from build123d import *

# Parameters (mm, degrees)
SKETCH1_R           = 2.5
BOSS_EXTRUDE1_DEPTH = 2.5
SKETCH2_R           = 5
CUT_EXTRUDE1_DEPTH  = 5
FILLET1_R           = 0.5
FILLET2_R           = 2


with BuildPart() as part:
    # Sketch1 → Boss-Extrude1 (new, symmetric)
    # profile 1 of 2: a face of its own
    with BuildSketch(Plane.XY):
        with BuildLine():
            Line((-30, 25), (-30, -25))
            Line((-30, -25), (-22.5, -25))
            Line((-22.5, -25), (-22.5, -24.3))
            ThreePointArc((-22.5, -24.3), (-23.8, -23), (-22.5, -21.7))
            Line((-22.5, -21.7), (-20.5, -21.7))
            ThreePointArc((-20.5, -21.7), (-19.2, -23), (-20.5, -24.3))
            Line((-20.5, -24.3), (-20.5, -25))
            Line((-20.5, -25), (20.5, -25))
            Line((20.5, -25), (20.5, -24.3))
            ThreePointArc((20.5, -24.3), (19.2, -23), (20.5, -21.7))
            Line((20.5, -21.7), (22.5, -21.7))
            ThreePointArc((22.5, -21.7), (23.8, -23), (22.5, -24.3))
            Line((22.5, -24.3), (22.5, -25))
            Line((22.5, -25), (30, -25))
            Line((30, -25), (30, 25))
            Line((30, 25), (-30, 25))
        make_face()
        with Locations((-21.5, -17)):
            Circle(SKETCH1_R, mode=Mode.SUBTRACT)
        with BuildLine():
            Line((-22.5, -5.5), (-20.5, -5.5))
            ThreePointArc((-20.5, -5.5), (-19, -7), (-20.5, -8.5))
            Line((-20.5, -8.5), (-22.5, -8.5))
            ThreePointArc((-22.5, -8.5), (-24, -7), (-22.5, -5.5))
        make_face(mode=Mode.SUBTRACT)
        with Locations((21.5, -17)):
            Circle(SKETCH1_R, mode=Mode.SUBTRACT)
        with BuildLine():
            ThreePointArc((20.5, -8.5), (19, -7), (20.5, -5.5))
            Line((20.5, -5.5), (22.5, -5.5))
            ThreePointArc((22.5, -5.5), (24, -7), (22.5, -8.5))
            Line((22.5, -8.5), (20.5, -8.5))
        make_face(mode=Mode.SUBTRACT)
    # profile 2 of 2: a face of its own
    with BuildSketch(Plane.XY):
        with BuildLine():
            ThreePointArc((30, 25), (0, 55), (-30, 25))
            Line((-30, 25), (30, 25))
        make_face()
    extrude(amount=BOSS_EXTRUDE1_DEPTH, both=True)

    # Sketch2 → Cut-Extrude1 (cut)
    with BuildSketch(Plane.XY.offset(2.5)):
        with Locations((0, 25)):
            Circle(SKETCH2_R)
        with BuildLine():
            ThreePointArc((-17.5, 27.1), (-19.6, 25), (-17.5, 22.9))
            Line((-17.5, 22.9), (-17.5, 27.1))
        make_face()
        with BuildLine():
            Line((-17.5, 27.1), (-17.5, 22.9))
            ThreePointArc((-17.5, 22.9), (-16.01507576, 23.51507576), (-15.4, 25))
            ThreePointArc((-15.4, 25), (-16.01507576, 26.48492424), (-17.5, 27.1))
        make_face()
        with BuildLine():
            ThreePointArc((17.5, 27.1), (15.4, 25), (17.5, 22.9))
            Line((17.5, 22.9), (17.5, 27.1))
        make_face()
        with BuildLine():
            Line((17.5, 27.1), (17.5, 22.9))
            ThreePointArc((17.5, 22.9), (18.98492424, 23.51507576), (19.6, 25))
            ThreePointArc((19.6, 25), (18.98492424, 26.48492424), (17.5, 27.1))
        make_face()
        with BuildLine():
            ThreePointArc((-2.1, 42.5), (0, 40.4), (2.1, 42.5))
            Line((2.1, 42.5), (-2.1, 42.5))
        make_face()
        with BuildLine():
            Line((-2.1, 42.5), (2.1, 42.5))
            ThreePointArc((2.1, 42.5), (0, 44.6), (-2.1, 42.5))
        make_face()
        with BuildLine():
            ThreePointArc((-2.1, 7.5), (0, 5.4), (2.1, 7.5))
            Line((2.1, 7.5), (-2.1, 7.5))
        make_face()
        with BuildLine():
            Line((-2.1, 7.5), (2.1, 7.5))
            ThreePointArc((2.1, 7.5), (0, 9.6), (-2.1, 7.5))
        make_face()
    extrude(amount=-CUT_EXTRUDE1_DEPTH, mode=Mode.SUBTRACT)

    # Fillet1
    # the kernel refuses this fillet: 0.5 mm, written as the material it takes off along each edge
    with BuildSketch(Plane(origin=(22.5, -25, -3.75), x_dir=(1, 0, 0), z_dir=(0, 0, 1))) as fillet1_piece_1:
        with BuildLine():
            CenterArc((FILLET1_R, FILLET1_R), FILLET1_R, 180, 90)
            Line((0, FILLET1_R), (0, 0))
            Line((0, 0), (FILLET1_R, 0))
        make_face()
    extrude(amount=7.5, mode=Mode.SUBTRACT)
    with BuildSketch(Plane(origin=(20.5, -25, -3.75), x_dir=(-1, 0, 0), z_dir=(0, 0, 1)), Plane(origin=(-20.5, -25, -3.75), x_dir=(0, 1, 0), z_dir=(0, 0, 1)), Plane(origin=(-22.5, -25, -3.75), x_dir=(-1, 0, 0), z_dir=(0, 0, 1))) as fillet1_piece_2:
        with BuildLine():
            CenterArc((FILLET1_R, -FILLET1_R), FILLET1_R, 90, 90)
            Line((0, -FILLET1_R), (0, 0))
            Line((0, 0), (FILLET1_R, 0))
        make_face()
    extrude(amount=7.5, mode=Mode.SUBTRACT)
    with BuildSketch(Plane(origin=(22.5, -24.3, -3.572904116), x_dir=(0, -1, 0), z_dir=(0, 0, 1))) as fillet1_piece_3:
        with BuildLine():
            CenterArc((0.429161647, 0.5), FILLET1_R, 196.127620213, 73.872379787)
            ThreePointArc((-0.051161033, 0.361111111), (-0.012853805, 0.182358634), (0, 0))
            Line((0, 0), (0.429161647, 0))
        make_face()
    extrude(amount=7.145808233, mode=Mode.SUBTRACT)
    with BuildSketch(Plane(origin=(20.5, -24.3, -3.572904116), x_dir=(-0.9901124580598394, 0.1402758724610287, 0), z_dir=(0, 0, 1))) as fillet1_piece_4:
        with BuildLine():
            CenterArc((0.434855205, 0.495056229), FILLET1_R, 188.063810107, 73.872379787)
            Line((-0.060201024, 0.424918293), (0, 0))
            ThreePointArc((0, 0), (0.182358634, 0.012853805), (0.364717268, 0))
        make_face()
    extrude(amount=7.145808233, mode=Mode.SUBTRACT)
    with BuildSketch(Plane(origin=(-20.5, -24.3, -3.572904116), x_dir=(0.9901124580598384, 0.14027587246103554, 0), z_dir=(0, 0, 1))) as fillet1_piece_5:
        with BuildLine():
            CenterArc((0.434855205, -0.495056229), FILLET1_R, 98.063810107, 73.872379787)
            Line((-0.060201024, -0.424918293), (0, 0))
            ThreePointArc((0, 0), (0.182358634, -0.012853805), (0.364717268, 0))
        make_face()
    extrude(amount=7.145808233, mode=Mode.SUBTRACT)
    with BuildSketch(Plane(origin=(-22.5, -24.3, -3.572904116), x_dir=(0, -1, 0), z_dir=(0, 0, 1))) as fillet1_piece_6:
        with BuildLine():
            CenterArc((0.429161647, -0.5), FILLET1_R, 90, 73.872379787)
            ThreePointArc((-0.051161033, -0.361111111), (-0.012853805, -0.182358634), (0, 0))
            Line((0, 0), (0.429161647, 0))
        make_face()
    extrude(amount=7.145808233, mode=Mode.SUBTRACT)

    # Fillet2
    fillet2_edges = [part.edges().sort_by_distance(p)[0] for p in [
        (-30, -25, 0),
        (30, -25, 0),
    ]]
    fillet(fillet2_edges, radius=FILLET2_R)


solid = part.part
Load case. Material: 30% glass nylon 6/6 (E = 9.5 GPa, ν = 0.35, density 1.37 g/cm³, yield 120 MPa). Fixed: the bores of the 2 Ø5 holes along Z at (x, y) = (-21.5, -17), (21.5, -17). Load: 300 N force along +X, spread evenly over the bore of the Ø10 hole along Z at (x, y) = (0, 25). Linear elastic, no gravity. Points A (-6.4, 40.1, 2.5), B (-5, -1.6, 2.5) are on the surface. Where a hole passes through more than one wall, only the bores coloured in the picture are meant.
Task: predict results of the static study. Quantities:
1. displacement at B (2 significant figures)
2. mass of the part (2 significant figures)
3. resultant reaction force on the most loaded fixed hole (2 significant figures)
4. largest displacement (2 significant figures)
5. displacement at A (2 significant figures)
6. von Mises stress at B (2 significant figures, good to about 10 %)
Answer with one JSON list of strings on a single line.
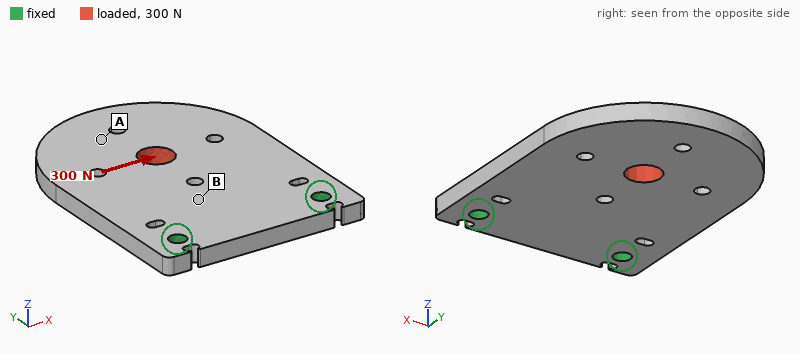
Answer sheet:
["8.6 µm", "29 g", "310 N", "41 µm", "36 µm", "2.5 MPa"]
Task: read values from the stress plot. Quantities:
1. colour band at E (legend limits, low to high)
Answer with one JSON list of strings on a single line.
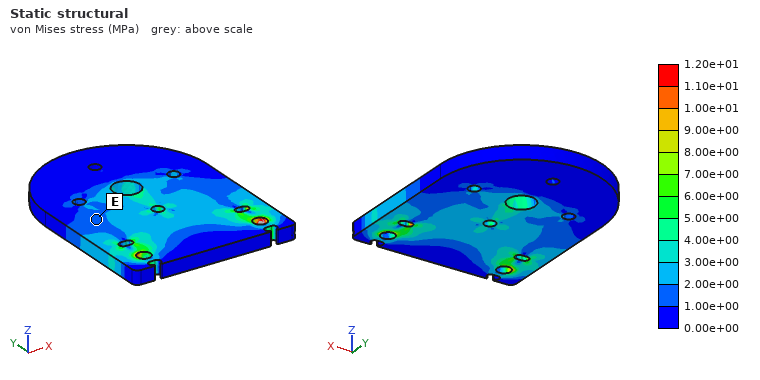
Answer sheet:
["1.00e+00 to 2.00e+00 MPa"]
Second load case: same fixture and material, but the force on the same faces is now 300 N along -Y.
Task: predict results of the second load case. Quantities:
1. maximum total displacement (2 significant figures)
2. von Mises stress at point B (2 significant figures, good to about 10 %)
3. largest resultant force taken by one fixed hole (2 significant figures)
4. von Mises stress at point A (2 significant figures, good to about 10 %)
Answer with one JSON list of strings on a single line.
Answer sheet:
["9.7 µm", "0.88 MPa", "150 N", "0.63 MPa"]
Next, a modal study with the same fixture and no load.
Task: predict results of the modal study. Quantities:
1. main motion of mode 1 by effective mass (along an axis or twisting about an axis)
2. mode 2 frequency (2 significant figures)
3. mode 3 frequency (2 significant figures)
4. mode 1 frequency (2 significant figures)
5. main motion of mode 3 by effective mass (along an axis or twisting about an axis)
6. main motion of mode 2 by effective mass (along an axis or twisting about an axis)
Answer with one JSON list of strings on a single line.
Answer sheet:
["along Z", "1400 Hz", "2500 Hz", "440 Hz", "along Z", "twisting about Y"]
